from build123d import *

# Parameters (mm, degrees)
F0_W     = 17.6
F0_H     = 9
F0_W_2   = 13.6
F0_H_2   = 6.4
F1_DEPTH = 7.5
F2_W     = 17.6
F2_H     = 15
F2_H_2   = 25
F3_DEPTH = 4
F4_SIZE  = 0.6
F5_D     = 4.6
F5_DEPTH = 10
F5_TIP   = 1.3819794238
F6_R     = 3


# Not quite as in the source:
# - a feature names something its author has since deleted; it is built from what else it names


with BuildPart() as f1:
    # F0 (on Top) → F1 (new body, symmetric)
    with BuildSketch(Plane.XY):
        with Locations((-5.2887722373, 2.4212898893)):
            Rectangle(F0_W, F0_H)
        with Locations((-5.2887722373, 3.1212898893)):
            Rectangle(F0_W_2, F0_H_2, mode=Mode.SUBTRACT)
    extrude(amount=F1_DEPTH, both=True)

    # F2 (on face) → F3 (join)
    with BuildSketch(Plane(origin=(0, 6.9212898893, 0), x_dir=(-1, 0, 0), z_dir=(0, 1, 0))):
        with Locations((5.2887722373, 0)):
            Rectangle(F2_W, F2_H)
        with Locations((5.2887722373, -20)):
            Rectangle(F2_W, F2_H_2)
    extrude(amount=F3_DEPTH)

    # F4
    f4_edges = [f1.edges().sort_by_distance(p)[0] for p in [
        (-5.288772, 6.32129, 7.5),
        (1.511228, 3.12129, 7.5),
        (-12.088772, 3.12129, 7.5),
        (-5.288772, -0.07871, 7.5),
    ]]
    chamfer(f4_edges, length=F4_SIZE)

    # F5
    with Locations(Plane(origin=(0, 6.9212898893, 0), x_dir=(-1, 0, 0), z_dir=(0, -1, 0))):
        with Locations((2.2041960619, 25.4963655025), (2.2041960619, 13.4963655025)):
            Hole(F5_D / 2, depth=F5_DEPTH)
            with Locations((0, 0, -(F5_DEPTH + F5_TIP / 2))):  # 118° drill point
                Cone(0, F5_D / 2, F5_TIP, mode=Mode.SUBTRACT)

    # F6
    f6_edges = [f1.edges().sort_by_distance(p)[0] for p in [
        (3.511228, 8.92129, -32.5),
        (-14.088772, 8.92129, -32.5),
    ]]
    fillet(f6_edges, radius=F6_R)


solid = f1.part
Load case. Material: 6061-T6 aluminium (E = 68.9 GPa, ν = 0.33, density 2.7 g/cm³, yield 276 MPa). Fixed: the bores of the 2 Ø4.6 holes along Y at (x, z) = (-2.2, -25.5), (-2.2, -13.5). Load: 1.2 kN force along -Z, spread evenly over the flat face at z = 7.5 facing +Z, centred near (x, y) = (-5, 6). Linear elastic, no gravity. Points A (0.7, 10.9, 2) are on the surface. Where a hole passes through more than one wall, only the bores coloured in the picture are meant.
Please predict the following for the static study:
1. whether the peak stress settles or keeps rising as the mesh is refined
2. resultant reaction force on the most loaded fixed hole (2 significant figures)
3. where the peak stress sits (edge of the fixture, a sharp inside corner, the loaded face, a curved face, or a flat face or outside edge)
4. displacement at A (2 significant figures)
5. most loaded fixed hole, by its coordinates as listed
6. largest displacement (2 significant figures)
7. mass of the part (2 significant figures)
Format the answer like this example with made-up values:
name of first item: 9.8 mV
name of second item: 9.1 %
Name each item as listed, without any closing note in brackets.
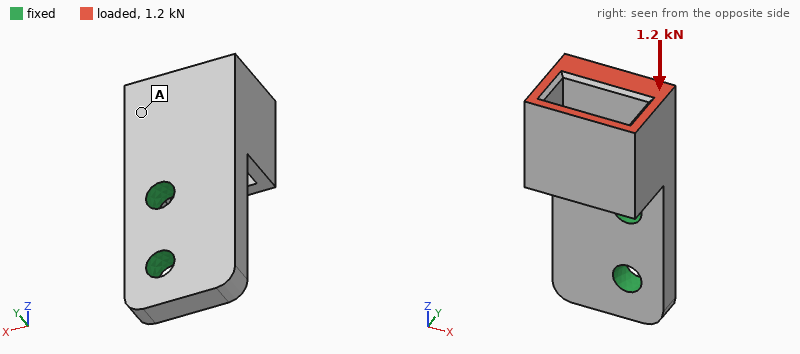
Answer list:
whether the peak stress settles or keeps rising as the mesh is refined: keeps rising
resultant reaction force on the most loaded fixed hole: 980 N
where the peak stress sits: edge of the fixture
displacement at A: 0.051 mm
most loaded fixed hole, by its coordinates as listed: (-2.2, -13.5)
largest displacement: 0.10 mm
mass of the part: 10 g
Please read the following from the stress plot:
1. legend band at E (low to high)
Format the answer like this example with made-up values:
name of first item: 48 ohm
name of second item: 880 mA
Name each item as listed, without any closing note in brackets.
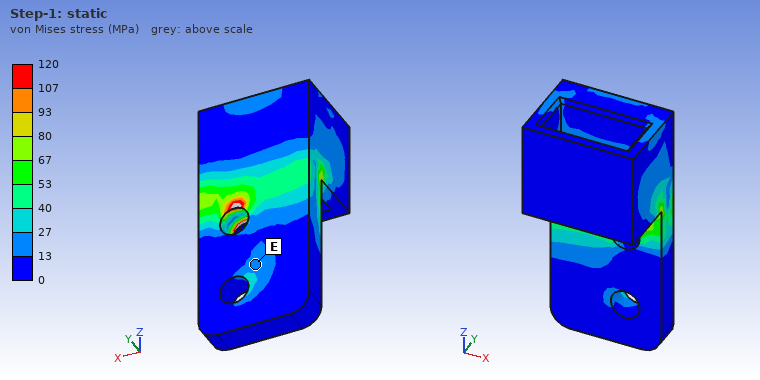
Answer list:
legend band at E: 13 to 27 MPa
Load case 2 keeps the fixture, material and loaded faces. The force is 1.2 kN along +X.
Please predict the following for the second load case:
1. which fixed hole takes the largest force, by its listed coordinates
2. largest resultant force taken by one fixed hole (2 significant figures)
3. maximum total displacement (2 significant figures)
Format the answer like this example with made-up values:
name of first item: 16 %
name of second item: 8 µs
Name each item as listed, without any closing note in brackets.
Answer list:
which fixed hole takes the largest force, by its listed coordinates: (-2.2, -13.5)
largest resultant force taken by one fixed hole: 2.4 kN
maximum total displacement: 0.12 mm
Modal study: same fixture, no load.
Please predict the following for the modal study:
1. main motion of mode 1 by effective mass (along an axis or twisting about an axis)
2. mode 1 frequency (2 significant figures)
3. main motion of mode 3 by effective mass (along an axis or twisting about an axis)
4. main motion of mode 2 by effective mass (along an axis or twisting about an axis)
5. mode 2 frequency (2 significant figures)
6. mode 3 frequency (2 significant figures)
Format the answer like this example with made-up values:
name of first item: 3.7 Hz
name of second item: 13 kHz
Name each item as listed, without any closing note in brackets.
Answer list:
main motion of mode 1 by effective mass: along Y
mode 1 frequency: 5000 Hz
main motion of mode 3 by effective mass: along X
main motion of mode 2 by effective mass: along X
mode 2 frequency: 8100 Hz
mode 3 frequency: 14 kHz
